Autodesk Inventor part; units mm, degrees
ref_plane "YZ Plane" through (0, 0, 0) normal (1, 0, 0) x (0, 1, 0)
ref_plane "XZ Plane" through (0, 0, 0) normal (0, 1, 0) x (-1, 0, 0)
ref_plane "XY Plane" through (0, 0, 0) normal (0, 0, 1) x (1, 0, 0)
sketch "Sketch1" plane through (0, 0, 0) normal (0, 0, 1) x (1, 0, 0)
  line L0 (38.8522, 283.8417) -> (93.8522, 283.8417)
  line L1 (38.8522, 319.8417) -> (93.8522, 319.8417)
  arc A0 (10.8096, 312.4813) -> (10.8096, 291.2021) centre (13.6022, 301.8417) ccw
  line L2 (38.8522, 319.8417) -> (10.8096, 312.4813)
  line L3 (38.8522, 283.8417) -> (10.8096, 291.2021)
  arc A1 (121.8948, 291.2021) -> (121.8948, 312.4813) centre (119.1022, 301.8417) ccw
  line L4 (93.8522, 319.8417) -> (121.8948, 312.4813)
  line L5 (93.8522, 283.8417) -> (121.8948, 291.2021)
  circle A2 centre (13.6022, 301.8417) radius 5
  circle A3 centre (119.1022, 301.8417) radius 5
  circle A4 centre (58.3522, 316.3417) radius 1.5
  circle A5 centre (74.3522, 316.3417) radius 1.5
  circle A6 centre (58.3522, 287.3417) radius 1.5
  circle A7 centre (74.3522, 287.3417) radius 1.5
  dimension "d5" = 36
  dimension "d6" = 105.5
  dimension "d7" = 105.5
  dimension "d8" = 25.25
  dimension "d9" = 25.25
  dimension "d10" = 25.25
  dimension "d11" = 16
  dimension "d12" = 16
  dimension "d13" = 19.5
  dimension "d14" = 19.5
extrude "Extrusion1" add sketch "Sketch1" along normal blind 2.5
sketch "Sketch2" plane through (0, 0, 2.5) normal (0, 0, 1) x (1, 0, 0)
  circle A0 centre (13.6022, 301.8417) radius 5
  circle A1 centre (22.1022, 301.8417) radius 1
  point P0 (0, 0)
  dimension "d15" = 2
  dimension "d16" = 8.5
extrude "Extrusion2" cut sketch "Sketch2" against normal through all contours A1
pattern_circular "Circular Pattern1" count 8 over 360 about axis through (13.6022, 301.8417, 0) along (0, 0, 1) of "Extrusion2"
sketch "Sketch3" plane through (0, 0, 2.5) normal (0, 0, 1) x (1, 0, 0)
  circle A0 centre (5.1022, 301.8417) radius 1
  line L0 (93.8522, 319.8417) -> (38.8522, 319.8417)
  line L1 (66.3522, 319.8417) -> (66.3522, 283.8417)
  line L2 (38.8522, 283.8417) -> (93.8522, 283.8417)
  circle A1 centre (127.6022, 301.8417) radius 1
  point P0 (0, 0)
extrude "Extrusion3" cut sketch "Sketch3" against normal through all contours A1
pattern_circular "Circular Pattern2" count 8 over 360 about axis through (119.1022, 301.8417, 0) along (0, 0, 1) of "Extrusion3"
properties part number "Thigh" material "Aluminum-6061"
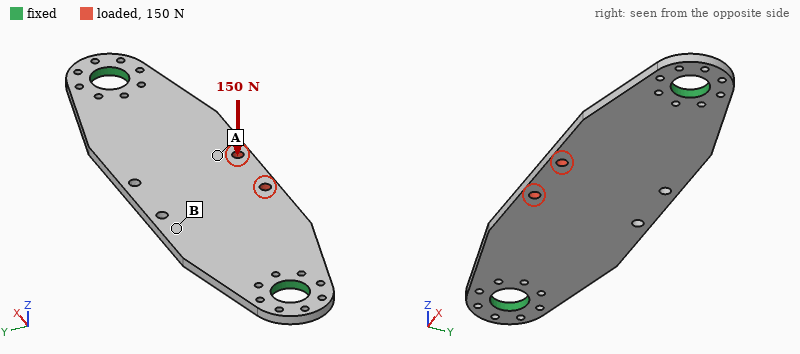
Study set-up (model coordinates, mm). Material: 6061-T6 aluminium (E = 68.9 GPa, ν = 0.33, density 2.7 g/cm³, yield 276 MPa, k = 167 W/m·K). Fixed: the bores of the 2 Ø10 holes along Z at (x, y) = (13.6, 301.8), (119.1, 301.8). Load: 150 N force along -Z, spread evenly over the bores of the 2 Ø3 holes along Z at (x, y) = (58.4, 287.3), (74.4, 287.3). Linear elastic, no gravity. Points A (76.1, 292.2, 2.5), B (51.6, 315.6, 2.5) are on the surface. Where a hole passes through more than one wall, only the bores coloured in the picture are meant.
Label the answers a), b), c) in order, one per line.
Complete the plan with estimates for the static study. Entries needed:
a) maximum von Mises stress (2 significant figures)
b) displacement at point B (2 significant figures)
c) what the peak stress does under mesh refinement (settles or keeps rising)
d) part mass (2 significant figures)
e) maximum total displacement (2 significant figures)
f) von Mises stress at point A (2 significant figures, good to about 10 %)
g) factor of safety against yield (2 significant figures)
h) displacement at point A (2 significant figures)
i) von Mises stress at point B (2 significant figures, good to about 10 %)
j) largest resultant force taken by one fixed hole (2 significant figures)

a) 170 MPa
b) 0.11 mm
c) settles
d) 24 g
e) 0.46 mm
f) 54 MPa
g) 1.6
h) 0.33 mm
i) 19 MPa
j) 75 N
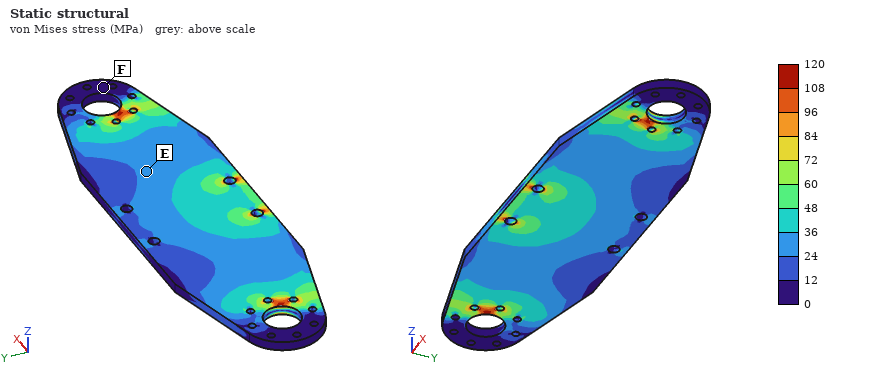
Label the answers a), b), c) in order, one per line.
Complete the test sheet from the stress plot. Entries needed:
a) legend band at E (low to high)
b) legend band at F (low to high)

a) 24 to 36 MPa
b) 0 to 12 MPa
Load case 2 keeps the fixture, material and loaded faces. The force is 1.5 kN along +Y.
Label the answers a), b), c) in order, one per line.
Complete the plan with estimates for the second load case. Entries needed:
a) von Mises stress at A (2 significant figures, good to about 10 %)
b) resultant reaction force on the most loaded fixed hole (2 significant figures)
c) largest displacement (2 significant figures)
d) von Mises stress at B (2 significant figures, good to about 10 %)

a) 29 MPa
b) 750 N
c) 50 µm
d) 22 MPa
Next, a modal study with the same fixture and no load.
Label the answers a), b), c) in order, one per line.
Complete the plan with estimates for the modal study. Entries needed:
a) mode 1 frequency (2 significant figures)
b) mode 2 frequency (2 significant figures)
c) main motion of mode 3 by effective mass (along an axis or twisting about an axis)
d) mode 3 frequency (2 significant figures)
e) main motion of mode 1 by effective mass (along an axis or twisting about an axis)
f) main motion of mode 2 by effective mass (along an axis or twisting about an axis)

a) 1200 Hz
b) 2100 Hz
c) twisting about Y
d) 3300 Hz
e) along Z
f) twisting about X
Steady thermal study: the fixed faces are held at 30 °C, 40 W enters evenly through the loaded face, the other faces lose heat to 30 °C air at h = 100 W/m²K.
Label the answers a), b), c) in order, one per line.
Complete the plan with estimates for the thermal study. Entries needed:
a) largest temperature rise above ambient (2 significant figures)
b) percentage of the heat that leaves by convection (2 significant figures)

a) 70 K
b) 47 %
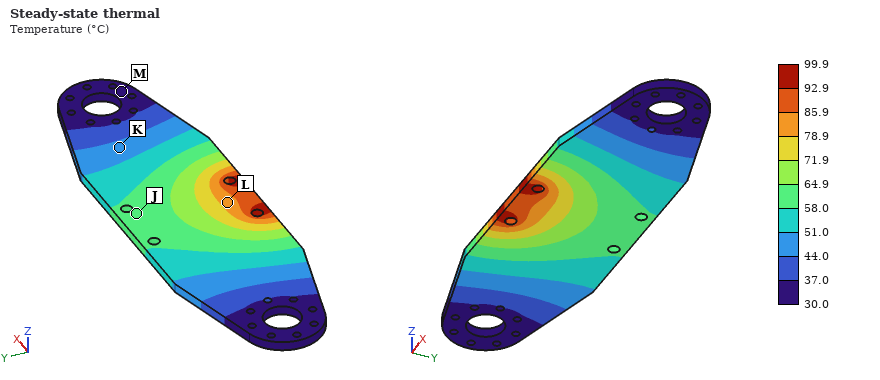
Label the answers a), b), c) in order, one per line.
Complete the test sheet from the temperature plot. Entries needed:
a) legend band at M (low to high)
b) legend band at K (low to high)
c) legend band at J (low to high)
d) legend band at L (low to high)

a) 30.0 to 37.0 °C
b) 44.0 to 51.0 °C
c) 58.0 to 64.9 °C
d) 78.9 to 85.9 °C
